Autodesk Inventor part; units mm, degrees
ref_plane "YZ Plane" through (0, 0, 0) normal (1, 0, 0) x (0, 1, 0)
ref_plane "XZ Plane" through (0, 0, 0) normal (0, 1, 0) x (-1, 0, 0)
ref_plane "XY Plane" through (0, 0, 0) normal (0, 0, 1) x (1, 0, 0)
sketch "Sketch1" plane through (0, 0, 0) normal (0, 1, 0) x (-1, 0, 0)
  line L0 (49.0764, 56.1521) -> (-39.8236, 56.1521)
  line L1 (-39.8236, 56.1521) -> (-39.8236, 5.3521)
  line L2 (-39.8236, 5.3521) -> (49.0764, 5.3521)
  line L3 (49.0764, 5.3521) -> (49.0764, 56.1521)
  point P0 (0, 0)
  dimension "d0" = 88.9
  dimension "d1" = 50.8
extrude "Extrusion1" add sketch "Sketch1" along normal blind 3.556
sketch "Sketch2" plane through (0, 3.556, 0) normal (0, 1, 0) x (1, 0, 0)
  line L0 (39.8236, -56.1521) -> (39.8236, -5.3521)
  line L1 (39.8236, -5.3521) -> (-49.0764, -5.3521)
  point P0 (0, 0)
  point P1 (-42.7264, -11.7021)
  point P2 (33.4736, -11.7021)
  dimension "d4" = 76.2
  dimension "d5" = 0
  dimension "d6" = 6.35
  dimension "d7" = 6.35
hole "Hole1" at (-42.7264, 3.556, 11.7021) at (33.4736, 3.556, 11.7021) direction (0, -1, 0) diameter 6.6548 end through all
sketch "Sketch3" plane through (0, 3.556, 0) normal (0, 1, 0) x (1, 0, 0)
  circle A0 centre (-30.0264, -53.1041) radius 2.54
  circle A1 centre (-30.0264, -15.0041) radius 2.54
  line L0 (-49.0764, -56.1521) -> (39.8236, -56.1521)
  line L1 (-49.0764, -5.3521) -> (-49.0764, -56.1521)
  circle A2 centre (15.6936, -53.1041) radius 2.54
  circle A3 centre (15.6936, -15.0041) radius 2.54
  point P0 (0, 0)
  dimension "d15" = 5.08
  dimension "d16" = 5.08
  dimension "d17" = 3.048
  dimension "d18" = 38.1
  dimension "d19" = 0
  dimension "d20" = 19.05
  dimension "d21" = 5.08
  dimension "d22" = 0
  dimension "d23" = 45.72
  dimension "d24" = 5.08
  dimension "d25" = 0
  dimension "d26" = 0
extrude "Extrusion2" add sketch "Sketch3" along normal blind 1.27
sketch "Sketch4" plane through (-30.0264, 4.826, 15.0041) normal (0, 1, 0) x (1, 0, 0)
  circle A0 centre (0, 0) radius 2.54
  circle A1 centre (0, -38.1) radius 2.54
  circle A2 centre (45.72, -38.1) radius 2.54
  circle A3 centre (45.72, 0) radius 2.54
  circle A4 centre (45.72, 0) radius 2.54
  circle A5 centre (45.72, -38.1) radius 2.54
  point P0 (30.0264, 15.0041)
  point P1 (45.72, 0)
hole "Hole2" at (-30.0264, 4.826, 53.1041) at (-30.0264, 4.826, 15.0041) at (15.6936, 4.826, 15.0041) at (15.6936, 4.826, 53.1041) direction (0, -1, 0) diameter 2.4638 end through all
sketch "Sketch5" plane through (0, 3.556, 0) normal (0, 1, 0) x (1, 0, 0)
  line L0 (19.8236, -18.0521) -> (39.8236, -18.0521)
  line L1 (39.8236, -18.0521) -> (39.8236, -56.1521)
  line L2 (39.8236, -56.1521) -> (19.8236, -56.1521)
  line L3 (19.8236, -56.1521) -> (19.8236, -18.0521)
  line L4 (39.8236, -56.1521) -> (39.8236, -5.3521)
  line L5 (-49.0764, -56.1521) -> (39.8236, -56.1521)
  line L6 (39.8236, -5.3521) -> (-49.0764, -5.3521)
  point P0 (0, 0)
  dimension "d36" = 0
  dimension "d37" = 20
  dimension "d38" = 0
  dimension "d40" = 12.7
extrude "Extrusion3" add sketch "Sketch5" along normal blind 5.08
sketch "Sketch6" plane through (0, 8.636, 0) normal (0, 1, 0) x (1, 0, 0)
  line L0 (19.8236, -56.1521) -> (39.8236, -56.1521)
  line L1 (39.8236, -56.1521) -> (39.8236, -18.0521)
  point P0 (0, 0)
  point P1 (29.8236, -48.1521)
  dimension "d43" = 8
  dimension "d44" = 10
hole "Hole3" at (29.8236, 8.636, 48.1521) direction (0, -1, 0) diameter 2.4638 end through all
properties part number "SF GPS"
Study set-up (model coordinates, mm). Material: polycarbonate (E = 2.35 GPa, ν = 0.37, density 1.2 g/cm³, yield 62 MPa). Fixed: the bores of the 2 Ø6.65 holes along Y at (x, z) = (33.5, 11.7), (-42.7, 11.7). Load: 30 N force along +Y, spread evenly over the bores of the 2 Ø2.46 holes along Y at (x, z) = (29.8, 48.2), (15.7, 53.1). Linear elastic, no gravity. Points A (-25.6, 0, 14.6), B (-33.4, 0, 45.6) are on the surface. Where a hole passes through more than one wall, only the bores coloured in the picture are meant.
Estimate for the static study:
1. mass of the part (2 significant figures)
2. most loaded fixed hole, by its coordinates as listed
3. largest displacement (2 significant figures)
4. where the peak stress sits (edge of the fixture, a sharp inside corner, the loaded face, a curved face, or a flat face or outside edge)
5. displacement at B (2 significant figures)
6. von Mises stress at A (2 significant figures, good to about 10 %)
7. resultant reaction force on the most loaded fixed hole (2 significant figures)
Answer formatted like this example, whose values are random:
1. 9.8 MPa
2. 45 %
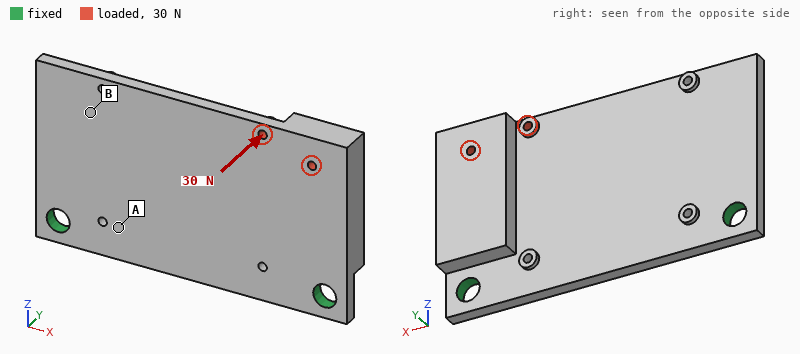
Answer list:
1. 24 g
2. (33.5, 11.7)
3. 1.1 mm
4. a flat face or outside edge
5. 0.43 mm
6. 2.8 MPa
7. 27 N
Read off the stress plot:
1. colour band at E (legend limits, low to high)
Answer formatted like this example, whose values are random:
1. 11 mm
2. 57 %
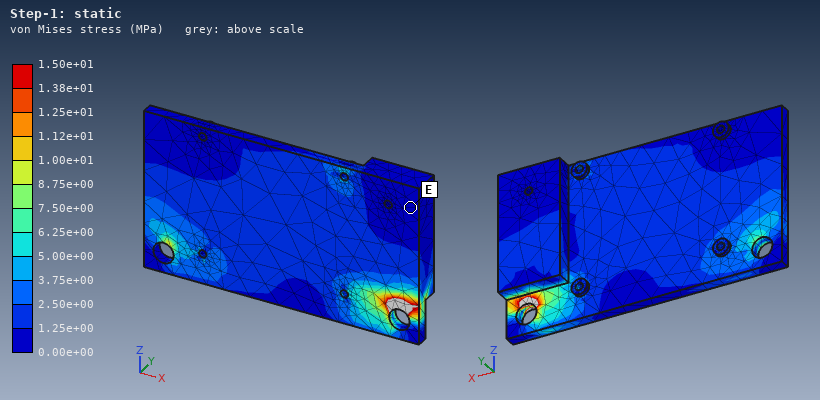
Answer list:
1. 0.00e+00 to 1.25e+00 MPa
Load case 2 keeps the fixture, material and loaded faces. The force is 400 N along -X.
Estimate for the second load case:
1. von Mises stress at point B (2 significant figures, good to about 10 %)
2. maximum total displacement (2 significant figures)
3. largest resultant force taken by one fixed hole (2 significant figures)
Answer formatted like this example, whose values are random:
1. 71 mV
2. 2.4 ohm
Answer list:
1. 1.0 MPa
2. 0.25 mm
3. 290 N
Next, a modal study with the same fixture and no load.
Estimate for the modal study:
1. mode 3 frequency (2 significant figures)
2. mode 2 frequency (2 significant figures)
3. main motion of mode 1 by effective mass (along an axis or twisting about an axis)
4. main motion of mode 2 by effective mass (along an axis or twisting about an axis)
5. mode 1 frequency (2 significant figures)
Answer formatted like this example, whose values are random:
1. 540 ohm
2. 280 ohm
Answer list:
1. 950 Hz
2. 620 Hz
3. along Y
4. twisting about Z
5. 320 Hz
